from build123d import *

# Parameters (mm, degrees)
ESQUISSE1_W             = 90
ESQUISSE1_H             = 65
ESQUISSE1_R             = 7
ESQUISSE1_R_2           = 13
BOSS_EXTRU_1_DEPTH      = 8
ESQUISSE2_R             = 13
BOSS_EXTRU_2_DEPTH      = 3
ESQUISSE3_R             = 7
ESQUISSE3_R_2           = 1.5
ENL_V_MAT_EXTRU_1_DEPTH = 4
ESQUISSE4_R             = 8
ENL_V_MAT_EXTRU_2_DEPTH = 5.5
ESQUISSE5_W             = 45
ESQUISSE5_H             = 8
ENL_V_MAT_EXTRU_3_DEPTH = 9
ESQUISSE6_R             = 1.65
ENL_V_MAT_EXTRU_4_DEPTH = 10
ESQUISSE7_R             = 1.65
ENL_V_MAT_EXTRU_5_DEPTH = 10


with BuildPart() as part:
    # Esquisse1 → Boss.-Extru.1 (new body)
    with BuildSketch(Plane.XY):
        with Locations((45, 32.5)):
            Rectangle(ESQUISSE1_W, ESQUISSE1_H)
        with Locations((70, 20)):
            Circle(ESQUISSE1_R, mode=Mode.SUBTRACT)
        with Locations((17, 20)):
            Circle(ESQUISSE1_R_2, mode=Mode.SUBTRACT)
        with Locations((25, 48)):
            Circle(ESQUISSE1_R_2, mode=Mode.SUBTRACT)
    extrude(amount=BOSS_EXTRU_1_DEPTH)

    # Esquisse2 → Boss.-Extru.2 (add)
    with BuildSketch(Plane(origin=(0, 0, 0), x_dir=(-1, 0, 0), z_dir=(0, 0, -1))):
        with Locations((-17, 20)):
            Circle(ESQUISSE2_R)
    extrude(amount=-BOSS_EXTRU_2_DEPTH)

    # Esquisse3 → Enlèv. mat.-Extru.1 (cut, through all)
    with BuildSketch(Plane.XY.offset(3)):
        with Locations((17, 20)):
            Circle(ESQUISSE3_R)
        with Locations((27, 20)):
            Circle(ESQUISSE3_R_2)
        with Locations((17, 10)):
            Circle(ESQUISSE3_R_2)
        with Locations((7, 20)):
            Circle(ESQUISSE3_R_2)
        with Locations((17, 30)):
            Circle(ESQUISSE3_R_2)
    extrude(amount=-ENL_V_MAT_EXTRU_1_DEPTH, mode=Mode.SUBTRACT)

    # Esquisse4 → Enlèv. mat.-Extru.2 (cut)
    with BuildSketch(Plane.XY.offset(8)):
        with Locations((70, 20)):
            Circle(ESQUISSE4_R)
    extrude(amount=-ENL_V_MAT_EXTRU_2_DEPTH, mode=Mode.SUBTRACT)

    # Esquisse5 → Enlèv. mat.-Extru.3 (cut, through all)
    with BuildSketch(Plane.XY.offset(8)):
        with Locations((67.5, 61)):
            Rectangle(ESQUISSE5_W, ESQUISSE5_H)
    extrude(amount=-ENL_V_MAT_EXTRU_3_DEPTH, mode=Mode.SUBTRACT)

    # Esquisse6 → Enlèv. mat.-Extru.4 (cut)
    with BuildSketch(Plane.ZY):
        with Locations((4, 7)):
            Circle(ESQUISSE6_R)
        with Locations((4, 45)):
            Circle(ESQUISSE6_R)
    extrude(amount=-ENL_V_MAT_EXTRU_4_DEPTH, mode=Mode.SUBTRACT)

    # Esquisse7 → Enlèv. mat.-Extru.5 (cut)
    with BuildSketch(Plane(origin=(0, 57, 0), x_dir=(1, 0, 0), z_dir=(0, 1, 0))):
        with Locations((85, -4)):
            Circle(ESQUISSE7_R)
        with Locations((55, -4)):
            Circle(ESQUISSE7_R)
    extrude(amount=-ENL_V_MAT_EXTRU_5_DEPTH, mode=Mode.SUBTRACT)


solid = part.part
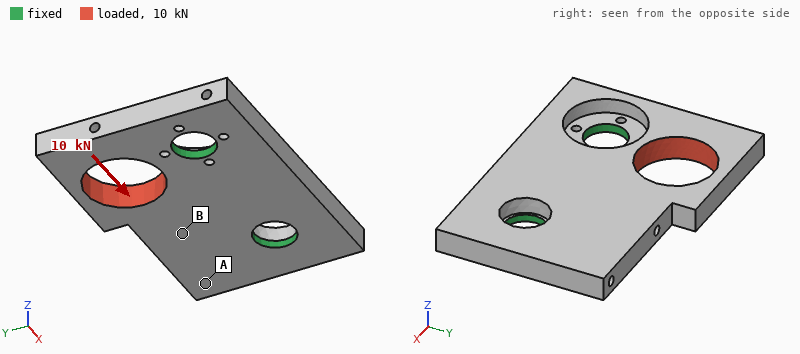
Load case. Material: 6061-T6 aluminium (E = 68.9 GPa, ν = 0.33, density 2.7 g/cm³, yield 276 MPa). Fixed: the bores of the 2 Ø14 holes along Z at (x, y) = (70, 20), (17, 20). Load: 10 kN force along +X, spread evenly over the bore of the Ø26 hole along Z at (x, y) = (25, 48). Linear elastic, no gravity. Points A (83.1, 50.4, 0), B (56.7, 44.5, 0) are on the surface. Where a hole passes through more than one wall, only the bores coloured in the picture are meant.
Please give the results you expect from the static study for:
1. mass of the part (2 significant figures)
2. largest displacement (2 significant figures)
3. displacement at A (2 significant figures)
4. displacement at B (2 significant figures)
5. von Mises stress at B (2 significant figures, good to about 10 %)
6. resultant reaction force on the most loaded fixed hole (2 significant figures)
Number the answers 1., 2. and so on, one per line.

1. 94 g
2. 100 µm
3. 30 µm
4. 26 µm
5. 43 MPa
6. 6.5 kN
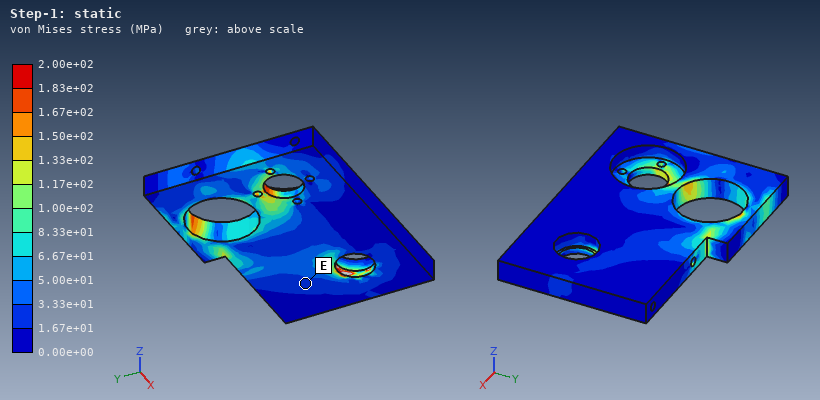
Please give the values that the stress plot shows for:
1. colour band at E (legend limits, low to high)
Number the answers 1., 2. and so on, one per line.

1. 1.67e+01 to 3.33e+01 MPa
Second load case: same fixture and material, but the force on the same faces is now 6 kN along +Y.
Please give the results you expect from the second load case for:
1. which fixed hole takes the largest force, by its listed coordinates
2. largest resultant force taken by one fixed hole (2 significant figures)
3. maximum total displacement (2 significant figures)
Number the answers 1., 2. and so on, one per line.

1. (17, 20)
2. 4.7 kN
3. 0.11 mm
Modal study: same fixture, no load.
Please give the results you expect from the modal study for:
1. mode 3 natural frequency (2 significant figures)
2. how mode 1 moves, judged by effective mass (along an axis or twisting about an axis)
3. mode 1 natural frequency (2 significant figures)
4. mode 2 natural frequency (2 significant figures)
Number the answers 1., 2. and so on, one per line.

1. 6900 Hz
2. along Z
3. 2600 Hz
4. 4200 Hz
